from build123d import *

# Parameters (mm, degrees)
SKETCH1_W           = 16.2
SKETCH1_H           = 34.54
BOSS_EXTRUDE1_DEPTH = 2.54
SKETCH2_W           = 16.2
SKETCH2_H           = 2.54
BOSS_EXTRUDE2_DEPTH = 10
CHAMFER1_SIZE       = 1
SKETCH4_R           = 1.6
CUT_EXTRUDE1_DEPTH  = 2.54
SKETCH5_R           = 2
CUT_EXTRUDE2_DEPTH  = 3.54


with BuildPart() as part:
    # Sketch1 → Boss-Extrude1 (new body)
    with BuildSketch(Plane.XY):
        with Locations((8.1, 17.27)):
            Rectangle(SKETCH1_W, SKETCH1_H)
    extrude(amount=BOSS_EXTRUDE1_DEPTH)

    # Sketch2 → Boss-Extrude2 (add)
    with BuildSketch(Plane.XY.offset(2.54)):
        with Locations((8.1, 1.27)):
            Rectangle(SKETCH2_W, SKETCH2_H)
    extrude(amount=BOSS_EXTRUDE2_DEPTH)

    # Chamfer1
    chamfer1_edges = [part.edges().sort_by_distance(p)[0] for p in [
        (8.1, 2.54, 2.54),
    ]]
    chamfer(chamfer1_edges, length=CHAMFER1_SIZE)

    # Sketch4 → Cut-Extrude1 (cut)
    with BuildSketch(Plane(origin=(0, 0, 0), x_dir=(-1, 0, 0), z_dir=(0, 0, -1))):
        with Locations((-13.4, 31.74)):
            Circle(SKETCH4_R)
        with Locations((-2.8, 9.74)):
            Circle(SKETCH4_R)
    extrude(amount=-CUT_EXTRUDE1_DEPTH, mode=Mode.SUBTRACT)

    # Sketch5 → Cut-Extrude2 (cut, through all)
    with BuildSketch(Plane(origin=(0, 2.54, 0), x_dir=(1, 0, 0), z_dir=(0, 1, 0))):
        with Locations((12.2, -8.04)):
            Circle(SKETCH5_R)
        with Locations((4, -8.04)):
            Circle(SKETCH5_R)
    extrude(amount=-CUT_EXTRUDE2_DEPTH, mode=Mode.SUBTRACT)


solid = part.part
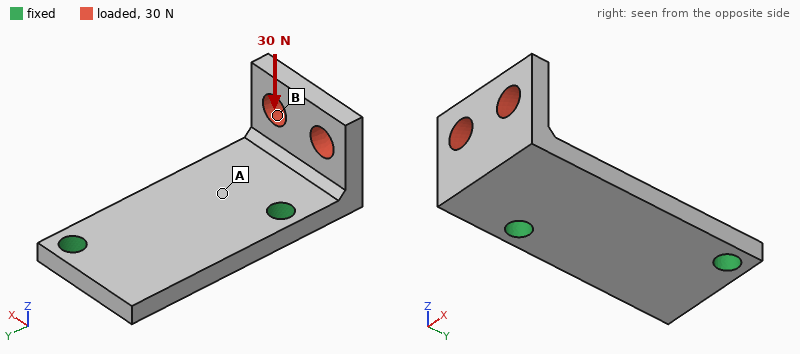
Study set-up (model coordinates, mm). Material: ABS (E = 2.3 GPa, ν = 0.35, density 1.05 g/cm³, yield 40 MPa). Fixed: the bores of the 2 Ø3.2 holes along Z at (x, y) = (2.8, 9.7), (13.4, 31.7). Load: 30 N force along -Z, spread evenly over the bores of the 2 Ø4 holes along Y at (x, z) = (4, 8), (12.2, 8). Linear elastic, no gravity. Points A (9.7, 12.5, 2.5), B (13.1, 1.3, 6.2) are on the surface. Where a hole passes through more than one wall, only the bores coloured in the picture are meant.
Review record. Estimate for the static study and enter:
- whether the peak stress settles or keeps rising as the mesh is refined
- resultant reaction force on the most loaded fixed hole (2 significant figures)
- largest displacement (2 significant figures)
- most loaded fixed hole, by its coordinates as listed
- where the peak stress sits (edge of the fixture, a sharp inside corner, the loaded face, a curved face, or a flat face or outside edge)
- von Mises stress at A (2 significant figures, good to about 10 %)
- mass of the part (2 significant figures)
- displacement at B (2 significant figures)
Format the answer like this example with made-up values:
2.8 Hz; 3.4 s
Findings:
keeps rising; 33 N; 0.46 mm; (2.8, 9.7); edge of the fixture; 5.6 MPa; 1.8 g; 0.30 mm
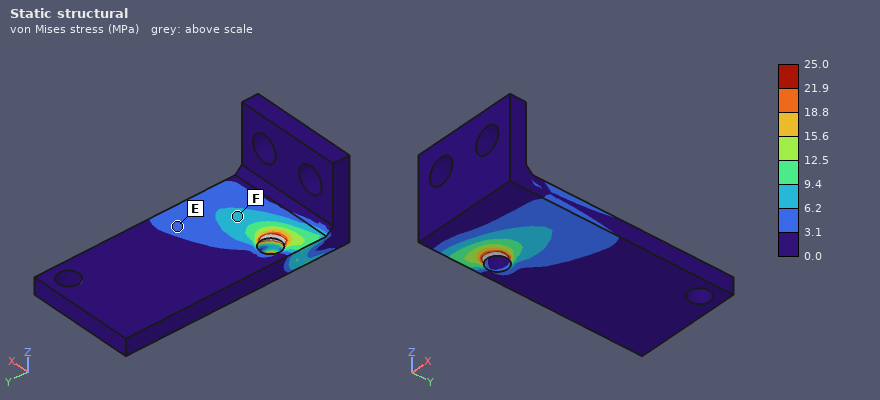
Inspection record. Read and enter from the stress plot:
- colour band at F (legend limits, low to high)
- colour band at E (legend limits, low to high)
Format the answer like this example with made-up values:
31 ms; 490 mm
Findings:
6.2 to 9.4 MPa; 3.1 to 6.2 MPa
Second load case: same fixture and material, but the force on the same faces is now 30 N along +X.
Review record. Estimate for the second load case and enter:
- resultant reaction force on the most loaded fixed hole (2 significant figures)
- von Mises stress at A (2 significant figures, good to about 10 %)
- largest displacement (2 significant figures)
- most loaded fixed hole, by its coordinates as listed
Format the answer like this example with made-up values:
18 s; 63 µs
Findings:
35 N; 4.5 MPa; 0.39 mm; (2.8, 9.7)
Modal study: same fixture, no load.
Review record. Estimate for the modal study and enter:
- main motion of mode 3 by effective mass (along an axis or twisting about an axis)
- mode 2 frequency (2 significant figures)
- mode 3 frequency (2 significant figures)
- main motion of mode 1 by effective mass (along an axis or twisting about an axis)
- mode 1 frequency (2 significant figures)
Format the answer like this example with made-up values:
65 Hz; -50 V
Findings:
along Z; 2700 Hz; 4300 Hz; along Z; 1900 Hz
